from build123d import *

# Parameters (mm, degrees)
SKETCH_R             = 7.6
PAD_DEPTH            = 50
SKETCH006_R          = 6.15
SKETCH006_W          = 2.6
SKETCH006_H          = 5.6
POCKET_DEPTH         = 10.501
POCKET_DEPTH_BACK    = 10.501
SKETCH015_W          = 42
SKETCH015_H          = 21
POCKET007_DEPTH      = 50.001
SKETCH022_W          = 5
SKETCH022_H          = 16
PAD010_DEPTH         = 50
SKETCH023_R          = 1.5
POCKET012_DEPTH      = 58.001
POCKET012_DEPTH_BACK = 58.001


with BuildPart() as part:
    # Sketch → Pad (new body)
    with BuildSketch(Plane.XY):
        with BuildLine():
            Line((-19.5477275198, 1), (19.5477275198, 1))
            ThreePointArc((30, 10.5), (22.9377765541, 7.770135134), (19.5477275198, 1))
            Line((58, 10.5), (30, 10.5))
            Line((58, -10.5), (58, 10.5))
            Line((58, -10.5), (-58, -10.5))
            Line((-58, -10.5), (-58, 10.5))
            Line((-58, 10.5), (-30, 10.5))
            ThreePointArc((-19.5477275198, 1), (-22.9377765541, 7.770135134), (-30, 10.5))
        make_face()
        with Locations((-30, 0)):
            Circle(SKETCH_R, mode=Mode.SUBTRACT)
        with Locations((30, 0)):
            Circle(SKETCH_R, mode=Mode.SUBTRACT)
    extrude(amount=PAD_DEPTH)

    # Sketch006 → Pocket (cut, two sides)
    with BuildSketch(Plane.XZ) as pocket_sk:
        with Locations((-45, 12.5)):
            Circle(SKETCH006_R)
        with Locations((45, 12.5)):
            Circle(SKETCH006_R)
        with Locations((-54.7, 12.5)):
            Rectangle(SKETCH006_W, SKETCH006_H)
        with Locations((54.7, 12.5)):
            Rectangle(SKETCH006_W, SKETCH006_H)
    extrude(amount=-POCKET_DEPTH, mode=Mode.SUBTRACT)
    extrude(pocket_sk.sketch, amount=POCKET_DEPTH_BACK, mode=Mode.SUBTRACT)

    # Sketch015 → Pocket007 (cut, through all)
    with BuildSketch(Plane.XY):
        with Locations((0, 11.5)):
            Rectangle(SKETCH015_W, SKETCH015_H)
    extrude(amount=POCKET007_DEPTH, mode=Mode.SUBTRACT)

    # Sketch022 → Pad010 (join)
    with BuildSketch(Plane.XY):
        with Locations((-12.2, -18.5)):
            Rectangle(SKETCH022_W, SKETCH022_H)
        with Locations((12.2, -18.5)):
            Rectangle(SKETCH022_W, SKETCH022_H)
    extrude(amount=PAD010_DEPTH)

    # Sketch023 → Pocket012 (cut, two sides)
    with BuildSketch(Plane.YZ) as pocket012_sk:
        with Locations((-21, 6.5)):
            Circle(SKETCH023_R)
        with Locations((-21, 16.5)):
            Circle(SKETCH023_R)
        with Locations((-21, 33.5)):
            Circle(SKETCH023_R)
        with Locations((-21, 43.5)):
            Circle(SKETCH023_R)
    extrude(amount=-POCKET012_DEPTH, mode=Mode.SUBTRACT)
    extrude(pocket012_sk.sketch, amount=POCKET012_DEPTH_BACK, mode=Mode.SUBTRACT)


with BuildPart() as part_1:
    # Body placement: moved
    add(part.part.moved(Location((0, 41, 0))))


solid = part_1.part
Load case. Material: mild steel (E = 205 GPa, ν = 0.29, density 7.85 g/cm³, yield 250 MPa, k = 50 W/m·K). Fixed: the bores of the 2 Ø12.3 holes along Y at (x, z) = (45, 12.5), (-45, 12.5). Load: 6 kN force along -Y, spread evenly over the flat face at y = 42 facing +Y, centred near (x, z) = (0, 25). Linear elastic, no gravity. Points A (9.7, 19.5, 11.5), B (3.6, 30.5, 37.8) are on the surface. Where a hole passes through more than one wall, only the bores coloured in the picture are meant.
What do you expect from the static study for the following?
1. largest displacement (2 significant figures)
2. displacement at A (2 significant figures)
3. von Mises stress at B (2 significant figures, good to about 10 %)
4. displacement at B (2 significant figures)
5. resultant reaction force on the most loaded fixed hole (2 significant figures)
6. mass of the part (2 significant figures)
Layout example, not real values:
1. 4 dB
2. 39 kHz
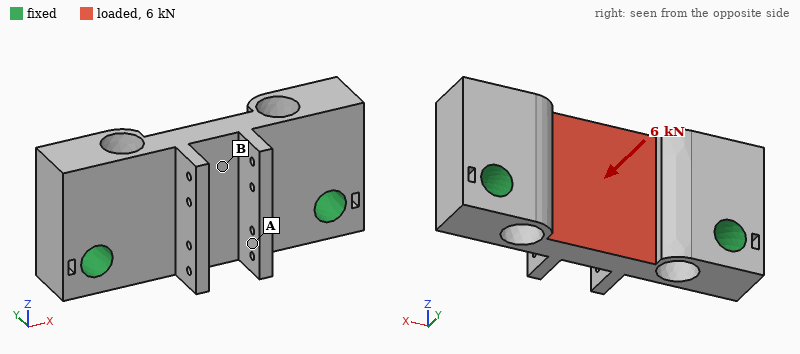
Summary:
1. 22 µm
2. 17 µm
3. 28 MPa
4. 20 µm
5. 3.0 kN
6. 660 g
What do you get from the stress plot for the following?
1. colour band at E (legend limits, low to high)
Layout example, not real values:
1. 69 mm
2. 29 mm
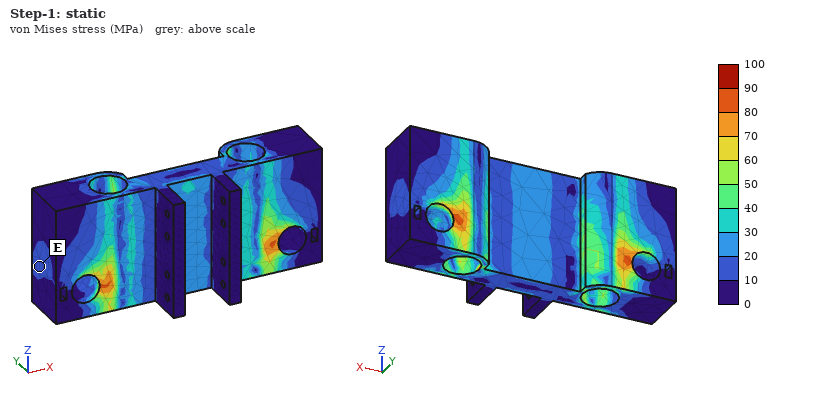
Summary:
1. 10 to 20 MPa
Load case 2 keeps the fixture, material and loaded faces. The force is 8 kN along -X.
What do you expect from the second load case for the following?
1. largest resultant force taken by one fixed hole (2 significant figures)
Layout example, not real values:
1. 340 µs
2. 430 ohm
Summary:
1. 4.2 kN
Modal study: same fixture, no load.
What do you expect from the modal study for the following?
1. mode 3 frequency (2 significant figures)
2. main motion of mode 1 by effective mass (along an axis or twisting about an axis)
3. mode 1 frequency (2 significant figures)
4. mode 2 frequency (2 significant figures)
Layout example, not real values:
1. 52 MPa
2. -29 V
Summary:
1. 9100 Hz
2. along Y
3. 5300 Hz
4. 7400 Hz
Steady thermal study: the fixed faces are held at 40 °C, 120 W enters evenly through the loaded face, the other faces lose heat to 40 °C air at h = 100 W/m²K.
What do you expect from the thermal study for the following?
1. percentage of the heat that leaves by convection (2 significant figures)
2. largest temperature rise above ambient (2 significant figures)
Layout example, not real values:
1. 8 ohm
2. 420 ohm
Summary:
1. 51 %
2. 69 K
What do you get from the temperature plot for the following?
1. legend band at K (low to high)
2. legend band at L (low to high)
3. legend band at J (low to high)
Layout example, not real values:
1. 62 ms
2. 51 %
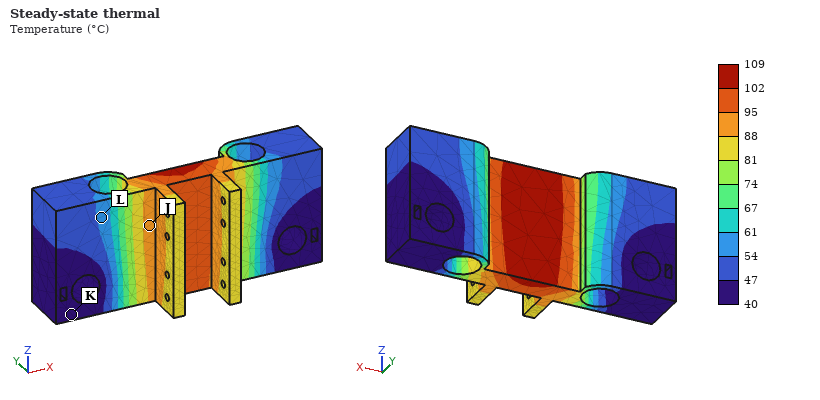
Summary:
1. 40 to 47 °C
2. 54 to 61 °C
3. 88 to 95 °C
